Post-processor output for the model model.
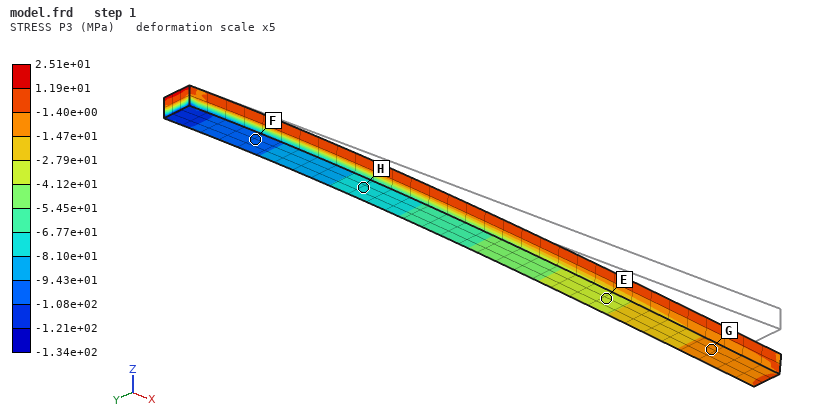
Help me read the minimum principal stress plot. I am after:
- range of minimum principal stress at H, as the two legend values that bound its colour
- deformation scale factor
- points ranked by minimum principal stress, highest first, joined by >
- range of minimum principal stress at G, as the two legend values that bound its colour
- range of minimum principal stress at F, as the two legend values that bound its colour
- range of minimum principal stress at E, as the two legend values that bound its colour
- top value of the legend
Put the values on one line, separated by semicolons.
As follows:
-8.10e+01 to -6.77e+01 MPa; 5; G > E > H > F; -1.47e+01 to -1.40e+00 MPa; -1.08e+02 to -9.43e+01 MPa; -4.12e+01 to -2.79e+01 MPa; 2.51e+01 MPa
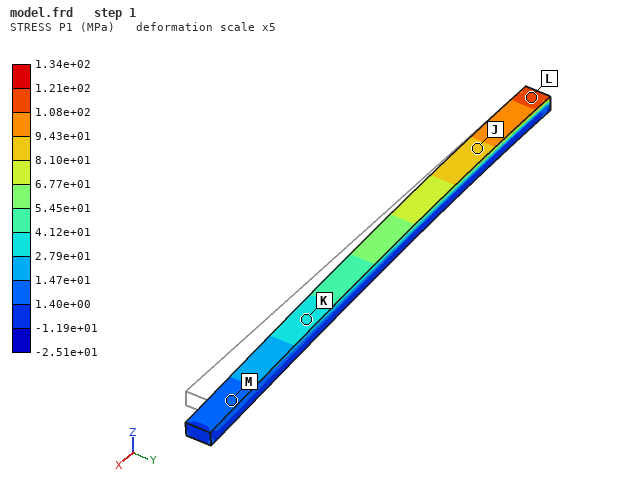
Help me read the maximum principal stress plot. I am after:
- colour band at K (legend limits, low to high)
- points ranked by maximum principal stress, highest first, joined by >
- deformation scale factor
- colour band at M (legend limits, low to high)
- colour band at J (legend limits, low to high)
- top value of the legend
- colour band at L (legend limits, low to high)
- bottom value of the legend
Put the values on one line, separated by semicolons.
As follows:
2.79e+01 to 4.12e+01 MPa; L > J > K > M; 5; 1.40e+00 to 1.47e+01 MPa; 8.10e+01 to 9.43e+01 MPa; 1.34e+02 MPa; 1.08e+02 to 1.21e+02 MPa; -2.51e+01 MPa
